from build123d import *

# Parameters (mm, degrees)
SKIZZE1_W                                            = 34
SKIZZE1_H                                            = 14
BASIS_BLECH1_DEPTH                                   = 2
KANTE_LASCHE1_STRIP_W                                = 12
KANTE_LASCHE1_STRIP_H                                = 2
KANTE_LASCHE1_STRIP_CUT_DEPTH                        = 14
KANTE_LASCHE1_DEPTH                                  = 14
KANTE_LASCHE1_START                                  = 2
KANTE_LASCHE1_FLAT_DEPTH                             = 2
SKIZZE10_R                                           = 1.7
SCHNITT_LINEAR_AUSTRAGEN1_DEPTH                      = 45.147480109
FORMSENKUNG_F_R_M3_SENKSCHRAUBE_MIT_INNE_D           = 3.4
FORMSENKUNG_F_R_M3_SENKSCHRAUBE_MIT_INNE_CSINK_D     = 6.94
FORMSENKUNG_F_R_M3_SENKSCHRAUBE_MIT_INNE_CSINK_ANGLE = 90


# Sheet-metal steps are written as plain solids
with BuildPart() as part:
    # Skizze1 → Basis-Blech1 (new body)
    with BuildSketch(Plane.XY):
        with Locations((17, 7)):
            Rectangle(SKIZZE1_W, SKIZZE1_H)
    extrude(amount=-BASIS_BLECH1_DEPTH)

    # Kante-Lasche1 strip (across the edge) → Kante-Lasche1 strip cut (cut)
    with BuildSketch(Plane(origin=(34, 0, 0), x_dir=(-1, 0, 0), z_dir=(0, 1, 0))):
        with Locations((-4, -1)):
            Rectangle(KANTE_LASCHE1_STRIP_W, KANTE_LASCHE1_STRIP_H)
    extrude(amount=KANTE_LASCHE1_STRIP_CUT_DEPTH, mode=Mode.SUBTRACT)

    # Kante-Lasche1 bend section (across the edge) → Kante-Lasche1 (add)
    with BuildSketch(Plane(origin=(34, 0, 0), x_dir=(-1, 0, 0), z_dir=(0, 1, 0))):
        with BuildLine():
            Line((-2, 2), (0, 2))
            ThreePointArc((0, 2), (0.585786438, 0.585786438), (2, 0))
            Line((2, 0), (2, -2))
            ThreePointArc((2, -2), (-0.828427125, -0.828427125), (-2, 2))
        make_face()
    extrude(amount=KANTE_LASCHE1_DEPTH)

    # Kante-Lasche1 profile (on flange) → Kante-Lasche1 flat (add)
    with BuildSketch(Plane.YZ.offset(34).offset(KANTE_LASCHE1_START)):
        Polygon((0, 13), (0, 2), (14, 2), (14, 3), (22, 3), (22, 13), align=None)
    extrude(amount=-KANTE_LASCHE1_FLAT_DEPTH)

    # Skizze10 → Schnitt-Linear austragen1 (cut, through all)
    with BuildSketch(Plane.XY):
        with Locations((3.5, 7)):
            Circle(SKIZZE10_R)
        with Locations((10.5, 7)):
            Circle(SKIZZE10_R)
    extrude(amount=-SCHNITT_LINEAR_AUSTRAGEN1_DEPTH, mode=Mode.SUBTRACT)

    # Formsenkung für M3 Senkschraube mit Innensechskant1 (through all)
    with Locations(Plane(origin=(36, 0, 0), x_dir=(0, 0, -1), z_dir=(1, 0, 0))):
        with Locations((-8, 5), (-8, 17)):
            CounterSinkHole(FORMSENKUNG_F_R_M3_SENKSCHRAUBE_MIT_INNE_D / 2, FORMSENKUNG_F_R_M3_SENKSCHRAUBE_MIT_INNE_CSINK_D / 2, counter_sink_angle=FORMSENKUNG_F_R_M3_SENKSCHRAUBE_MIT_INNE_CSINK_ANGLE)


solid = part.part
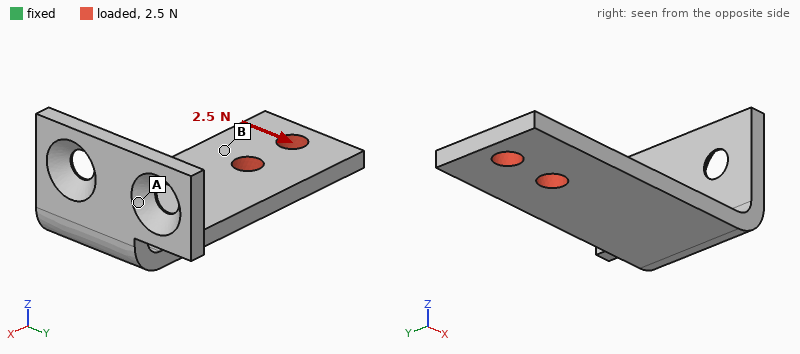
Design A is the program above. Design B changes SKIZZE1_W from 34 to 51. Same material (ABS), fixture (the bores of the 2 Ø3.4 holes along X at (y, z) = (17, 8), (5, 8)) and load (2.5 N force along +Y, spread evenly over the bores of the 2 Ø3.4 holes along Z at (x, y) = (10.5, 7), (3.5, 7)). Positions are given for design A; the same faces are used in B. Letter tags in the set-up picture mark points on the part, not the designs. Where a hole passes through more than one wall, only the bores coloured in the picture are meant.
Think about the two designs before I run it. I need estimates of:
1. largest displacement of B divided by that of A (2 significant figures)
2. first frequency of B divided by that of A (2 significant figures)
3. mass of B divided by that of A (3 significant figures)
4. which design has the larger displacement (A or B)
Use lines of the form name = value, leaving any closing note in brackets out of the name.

largest displacement of B divided by that of A = 1.2
first frequency of B divided by that of A = 0.68
mass of B divided by that of A = 1.17
which design has the larger displacement = B
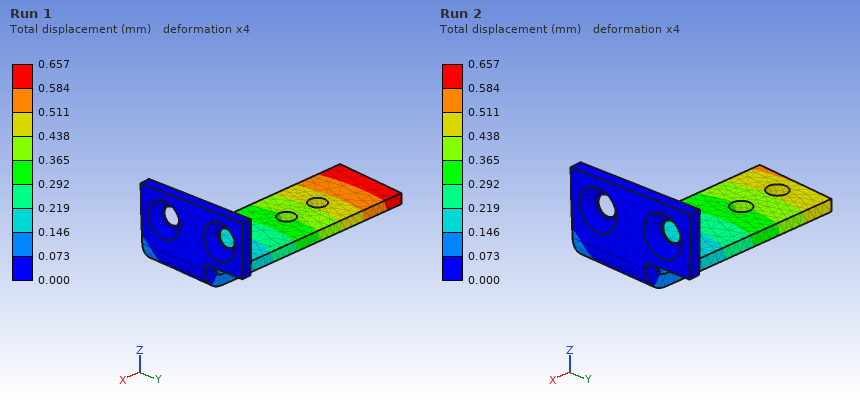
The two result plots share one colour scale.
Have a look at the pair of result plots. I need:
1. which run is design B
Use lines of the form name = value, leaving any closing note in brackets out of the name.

which run is design B = Run 1
